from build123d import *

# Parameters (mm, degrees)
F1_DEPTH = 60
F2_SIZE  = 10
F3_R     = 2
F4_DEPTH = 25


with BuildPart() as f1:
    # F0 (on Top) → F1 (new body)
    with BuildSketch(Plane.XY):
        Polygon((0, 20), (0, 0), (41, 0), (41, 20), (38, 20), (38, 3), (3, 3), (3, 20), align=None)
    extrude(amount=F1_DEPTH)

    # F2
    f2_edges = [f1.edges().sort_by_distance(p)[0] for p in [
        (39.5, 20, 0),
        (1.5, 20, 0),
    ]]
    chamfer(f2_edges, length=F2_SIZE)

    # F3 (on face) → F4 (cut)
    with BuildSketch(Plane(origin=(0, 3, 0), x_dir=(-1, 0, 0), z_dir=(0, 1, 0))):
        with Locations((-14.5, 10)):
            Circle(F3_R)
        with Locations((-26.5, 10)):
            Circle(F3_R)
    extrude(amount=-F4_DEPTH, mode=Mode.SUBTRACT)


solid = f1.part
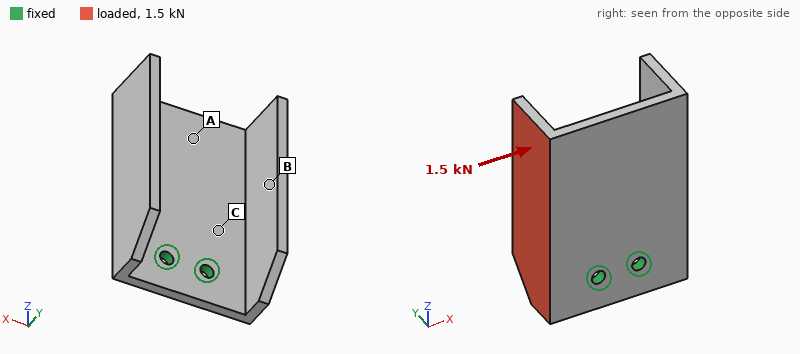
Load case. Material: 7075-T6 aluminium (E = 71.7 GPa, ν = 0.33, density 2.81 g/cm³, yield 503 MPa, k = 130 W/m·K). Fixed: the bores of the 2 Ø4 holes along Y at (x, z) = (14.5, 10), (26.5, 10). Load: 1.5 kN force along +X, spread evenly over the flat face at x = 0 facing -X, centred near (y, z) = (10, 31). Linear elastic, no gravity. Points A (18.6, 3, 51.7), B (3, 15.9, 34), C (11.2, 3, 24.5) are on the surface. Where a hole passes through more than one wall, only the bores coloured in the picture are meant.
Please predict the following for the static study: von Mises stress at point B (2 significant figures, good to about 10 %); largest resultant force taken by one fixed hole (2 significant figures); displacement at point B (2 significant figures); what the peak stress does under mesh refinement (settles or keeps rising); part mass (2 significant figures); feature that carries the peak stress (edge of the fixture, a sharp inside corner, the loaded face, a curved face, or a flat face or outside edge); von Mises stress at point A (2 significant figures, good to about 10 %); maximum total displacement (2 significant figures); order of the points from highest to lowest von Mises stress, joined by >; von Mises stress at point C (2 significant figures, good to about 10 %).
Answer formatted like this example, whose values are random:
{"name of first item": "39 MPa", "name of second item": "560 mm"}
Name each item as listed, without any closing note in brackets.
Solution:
{"von Mises stress at point B": "27 MPa", "largest resultant force taken by one fixed hole": "2.3 kN", "displacement at point B": "0.53 mm", "what the peak stress does under mesh refinement": "keeps rising", "part mass": "37 g", "feature that carries the peak stress": "edge of the fixture", "von Mises stress at point A": "86 MPa", "maximum total displacement": "0.87 mm", "order of the points from highest to lowest von Mises stress, joined by >": "C > A > B", "von Mises stress at point C": "140 MPa"}
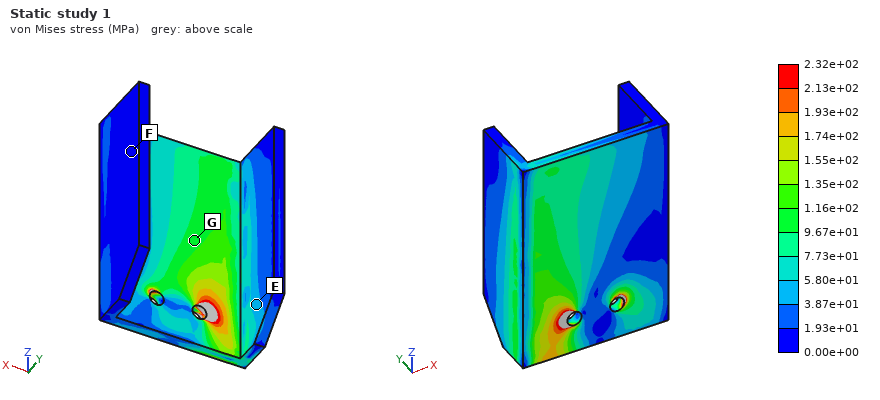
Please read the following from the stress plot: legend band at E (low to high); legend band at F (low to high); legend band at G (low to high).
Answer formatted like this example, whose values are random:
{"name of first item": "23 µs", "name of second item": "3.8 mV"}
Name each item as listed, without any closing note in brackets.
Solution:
{"legend band at E": "3.87e+01 to 5.80e+01 MPa", "legend band at F": "0.00e+00 to 1.93e+01 MPa", "legend band at G": "9.67e+01 to 1.16e+02 MPa"}
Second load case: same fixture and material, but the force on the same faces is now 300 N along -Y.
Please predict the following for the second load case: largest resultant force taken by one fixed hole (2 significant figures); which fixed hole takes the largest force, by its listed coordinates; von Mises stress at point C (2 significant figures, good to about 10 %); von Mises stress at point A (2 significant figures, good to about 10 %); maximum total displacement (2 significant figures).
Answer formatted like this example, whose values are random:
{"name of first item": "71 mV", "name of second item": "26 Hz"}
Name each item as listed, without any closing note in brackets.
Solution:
{"largest resultant force taken by one fixed hole": "420 N", "which fixed hole takes the largest force, by its listed coordinates": "(14.5, 10)", "von Mises stress at point C": "38 MPa", "von Mises stress at point A": "25 MPa", "maximum total displacement": "0.49 mm"}
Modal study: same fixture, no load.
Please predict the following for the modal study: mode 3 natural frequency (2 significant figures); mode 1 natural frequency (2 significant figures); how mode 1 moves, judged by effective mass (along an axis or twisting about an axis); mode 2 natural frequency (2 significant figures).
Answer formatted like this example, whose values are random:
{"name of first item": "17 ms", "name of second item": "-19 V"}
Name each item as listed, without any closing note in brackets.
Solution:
{"mode 3 natural frequency": "3300 Hz", "mode 1 natural frequency": "1100 Hz", "how mode 1 moves, judged by effective mass": "along Y", "mode 2 natural frequency": "1500 Hz"}
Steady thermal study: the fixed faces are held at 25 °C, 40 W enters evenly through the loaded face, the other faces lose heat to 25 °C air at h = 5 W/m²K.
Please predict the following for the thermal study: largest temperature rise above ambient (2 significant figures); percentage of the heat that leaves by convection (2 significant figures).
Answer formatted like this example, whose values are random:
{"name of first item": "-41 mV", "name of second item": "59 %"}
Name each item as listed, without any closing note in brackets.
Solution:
{"largest temperature rise above ambient": "73 K", "percentage of the heat that leaves by convection": "3.3 %"}
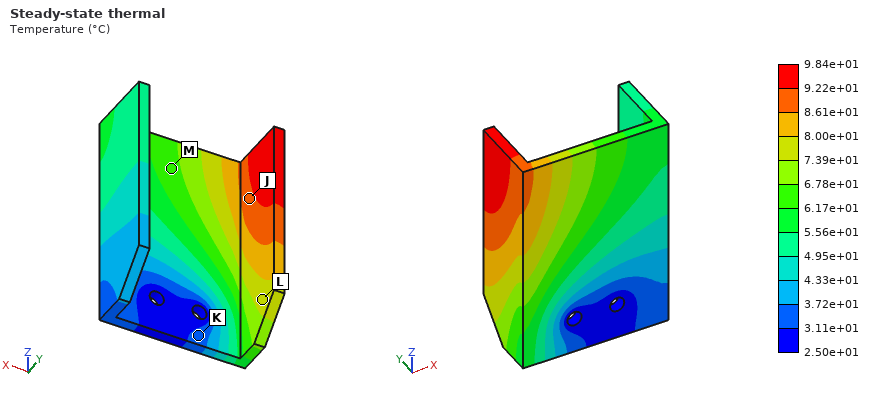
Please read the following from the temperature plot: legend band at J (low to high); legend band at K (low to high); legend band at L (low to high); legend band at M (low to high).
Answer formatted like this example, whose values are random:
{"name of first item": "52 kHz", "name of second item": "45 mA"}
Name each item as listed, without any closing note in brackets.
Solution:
{"legend band at J": "8.61e+01 to 9.22e+01 °C", "legend band at K": "3.11e+01 to 3.72e+01 °C", "legend band at L": "7.39e+01 to 8.00e+01 °C", "legend band at M": "6.17e+01 to 6.78e+01 °C"}
